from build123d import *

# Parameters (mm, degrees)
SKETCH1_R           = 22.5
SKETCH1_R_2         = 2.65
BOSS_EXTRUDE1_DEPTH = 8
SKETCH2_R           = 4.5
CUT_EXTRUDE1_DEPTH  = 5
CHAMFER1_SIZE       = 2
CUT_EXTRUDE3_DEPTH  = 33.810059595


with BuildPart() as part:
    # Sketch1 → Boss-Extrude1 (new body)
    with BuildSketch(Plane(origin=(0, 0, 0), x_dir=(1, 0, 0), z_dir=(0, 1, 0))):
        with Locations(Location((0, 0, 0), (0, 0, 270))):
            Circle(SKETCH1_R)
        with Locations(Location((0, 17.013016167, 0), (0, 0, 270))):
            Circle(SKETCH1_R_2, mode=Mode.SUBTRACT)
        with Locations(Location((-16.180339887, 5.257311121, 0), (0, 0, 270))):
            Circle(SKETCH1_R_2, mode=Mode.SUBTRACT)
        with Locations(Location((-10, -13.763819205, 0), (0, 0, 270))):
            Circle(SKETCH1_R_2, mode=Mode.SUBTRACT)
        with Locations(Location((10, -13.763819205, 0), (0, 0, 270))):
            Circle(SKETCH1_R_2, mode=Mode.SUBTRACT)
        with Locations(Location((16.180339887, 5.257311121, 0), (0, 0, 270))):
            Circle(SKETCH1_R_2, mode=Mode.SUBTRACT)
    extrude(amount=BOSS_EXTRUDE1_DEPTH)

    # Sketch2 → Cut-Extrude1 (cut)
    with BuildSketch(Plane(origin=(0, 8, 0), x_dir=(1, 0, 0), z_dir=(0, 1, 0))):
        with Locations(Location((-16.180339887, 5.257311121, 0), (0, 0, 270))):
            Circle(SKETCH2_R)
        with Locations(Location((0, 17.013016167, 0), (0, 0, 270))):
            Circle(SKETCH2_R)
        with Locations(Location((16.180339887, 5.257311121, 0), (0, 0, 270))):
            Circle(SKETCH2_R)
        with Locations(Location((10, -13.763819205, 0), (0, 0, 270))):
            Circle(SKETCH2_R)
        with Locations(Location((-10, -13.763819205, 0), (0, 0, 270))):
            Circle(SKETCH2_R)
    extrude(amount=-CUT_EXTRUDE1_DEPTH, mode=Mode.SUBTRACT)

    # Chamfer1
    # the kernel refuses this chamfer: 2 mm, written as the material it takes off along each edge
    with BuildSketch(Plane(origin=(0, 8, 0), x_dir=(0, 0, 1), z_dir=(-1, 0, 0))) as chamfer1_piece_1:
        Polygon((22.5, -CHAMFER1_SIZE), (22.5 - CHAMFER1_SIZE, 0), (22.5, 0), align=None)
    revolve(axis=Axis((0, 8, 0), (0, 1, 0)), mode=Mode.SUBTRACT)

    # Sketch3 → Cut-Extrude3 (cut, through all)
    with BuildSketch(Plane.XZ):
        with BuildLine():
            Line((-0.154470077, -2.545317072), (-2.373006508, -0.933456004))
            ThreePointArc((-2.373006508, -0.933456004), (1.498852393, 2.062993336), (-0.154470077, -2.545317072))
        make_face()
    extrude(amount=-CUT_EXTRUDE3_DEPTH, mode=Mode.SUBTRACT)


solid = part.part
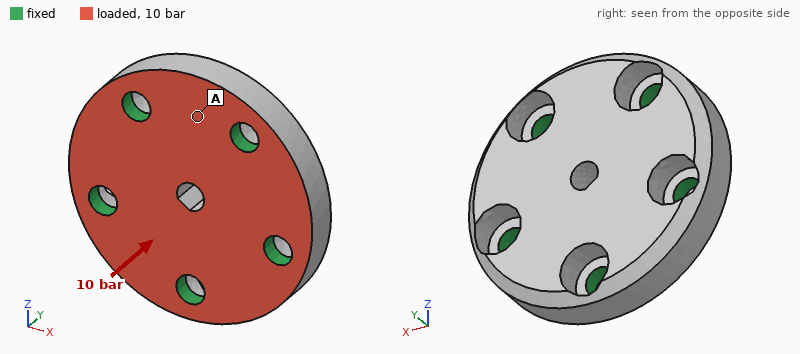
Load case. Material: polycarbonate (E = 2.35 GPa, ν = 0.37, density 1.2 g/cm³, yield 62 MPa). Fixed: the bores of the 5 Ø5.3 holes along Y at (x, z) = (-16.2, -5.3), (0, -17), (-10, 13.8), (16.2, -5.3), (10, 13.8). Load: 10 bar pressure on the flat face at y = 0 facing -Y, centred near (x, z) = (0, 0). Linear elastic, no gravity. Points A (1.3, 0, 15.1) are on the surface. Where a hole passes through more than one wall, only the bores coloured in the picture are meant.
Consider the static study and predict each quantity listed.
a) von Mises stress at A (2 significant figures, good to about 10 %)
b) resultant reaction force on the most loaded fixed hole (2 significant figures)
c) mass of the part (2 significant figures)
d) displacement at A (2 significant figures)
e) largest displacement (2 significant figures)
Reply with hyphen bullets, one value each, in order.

- 2.4 MPa
- 300 N
- 12 g
- 26 µm
- 41 µm
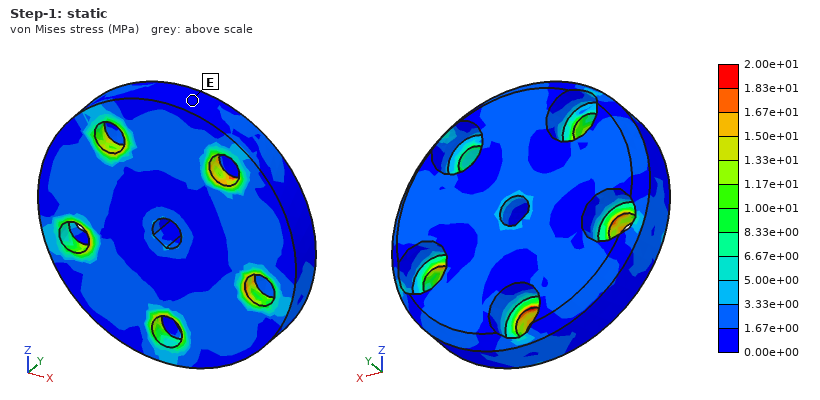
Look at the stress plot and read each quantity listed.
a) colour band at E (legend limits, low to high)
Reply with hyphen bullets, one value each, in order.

- 0.00e+00 to 1.67e+00 MPa
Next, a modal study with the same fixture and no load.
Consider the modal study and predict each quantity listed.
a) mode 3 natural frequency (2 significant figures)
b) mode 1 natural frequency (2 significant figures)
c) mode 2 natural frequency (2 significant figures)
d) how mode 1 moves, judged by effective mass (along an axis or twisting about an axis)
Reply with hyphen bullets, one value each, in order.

- 10 kHz
- 9500 Hz
- 10 kHz
- along Y
